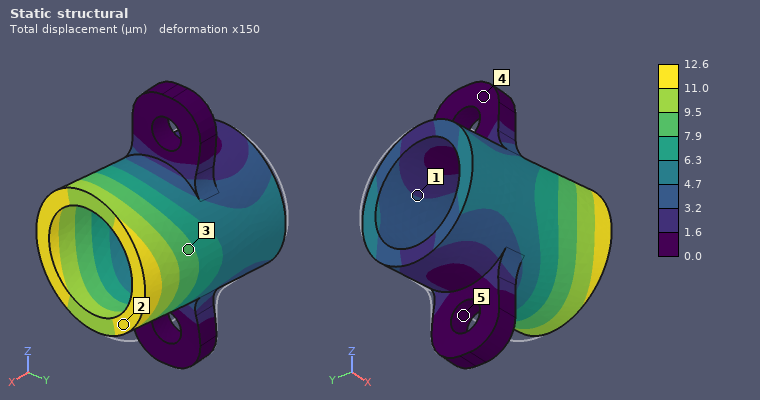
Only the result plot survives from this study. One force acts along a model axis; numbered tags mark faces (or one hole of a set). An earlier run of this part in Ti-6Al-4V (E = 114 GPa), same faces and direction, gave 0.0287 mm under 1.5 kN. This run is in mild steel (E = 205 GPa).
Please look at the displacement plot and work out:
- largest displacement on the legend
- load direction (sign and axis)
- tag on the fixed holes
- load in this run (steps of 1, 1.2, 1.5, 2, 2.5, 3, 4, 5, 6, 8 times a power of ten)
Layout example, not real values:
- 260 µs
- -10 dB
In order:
- 12.6 µm
- -Y
- 5
- 1.2 kN
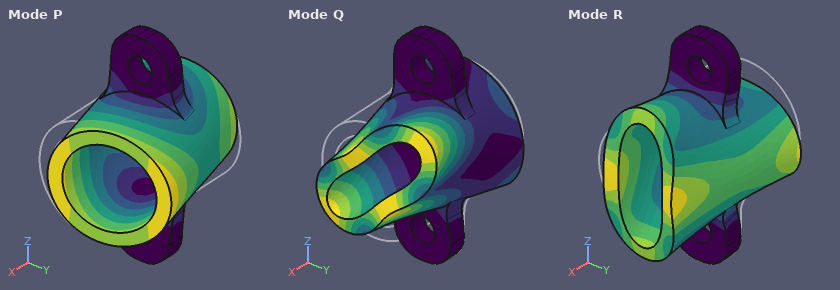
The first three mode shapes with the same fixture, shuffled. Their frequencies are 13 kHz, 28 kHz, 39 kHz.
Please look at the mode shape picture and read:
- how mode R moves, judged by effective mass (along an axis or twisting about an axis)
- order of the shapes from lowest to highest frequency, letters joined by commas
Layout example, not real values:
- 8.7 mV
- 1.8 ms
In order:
- along X
- P, R, Q
